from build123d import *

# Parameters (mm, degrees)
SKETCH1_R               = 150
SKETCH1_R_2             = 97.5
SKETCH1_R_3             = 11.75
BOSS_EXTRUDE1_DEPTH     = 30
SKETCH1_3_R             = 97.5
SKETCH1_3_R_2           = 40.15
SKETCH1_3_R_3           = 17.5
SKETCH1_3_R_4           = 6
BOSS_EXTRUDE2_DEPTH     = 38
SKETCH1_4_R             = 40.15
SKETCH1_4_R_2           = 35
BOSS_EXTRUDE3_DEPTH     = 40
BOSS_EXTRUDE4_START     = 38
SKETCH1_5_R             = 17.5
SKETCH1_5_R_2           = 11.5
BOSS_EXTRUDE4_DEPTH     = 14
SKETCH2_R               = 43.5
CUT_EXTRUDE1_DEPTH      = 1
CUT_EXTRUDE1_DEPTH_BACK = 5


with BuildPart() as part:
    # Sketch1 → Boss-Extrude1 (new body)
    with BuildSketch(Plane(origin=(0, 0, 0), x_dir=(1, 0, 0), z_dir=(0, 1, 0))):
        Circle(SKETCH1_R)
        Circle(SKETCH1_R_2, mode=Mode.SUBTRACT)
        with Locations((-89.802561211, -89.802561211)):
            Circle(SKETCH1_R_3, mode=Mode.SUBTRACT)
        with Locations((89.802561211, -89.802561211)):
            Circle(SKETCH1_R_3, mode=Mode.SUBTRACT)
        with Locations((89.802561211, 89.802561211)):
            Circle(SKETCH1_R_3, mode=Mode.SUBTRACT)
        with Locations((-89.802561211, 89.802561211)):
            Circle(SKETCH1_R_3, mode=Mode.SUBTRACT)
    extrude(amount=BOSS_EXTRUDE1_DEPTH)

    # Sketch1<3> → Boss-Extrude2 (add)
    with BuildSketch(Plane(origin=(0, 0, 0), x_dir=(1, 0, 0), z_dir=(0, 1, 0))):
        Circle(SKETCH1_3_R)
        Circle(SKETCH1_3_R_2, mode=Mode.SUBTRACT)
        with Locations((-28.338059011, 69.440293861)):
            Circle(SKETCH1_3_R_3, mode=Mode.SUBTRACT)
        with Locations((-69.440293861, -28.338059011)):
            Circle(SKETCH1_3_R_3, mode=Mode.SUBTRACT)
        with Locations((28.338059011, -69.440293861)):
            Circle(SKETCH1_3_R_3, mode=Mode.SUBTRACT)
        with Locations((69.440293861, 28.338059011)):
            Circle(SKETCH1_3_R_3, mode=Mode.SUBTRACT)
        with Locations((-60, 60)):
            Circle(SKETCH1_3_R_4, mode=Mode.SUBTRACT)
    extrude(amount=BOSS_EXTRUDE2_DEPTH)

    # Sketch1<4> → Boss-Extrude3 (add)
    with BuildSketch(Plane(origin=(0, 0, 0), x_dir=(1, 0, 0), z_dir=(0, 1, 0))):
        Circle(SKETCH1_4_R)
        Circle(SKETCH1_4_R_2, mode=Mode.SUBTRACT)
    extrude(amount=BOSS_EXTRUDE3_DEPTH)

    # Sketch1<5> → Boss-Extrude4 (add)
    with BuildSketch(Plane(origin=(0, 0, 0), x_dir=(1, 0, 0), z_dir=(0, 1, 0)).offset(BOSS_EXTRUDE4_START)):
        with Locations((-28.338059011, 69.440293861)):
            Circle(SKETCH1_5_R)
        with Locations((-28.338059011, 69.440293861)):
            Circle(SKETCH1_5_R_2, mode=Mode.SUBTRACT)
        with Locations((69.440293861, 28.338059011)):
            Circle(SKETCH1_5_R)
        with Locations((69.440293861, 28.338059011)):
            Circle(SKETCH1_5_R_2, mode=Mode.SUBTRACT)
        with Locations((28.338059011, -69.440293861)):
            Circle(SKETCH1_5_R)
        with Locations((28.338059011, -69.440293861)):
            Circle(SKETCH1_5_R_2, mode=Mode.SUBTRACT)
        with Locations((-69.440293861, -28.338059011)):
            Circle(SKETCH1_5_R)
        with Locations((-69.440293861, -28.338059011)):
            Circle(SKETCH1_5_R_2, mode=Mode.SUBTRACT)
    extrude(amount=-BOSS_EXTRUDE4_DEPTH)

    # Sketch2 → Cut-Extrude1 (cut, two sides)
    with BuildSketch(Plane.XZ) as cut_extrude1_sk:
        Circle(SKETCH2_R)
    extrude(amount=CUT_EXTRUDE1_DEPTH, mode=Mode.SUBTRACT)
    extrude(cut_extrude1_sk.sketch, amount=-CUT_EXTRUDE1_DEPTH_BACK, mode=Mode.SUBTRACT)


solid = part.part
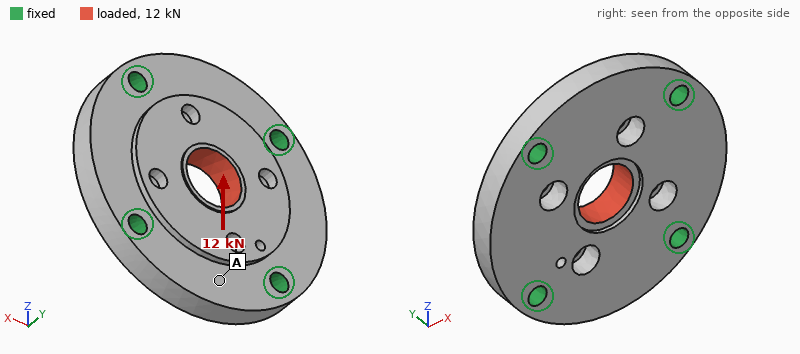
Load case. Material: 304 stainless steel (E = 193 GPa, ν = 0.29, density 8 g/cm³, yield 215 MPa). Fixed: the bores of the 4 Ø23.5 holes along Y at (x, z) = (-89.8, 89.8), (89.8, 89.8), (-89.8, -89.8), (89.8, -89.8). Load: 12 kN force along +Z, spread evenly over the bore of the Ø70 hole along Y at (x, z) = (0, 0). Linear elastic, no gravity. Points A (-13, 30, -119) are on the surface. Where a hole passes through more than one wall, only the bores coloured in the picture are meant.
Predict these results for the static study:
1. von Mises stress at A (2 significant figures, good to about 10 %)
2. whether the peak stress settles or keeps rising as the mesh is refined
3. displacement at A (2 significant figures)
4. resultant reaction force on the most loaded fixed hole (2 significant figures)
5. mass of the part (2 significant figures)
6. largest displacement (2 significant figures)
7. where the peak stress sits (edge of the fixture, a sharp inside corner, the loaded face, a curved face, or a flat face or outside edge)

0.80 MPa
keeps rising
0.75 µm
3.3 kN
16 kg
1.4 µm
edge of the fixture
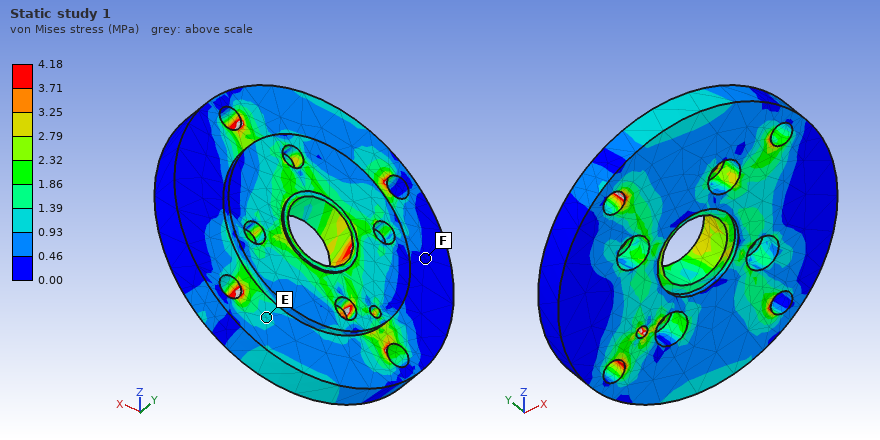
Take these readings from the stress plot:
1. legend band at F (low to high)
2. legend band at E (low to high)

0.00 to 0.46 MPa
0.93 to 1.39 MPa
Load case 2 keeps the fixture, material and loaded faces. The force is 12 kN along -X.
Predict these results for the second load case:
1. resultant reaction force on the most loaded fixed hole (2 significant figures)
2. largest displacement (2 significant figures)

3.3 kN
1.4 µm
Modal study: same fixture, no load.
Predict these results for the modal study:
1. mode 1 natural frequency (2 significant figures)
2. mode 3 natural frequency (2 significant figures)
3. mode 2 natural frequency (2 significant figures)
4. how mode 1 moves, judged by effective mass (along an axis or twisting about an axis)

3300 Hz
3800 Hz
3600 Hz
along Y
